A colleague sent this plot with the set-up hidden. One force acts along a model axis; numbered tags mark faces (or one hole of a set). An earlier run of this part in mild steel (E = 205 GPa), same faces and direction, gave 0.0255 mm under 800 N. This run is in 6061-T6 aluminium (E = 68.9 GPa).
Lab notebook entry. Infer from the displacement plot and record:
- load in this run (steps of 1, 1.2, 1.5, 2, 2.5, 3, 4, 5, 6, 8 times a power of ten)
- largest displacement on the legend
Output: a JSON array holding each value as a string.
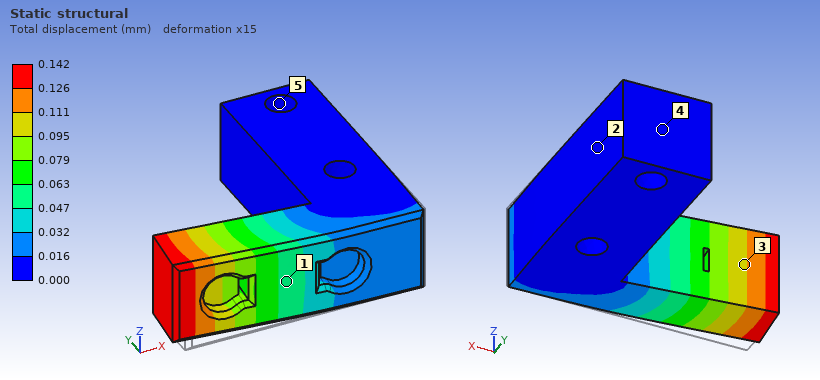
["1.5 kN", "0.142 mm"]
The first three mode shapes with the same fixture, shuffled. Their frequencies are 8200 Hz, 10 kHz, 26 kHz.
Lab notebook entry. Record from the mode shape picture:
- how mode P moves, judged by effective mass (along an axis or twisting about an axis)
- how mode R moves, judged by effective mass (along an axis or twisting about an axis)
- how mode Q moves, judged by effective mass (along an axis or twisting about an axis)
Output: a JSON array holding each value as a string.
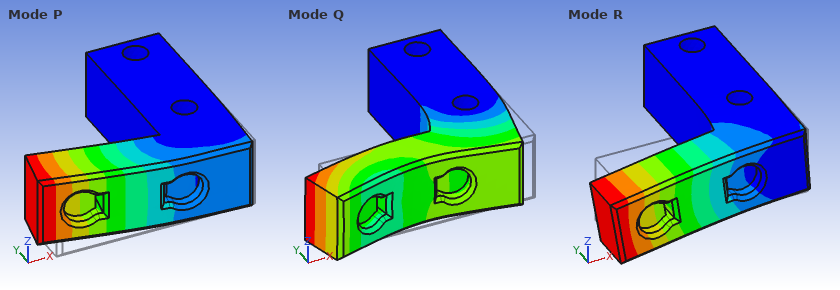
["along Y", "along Z", "along X"]
